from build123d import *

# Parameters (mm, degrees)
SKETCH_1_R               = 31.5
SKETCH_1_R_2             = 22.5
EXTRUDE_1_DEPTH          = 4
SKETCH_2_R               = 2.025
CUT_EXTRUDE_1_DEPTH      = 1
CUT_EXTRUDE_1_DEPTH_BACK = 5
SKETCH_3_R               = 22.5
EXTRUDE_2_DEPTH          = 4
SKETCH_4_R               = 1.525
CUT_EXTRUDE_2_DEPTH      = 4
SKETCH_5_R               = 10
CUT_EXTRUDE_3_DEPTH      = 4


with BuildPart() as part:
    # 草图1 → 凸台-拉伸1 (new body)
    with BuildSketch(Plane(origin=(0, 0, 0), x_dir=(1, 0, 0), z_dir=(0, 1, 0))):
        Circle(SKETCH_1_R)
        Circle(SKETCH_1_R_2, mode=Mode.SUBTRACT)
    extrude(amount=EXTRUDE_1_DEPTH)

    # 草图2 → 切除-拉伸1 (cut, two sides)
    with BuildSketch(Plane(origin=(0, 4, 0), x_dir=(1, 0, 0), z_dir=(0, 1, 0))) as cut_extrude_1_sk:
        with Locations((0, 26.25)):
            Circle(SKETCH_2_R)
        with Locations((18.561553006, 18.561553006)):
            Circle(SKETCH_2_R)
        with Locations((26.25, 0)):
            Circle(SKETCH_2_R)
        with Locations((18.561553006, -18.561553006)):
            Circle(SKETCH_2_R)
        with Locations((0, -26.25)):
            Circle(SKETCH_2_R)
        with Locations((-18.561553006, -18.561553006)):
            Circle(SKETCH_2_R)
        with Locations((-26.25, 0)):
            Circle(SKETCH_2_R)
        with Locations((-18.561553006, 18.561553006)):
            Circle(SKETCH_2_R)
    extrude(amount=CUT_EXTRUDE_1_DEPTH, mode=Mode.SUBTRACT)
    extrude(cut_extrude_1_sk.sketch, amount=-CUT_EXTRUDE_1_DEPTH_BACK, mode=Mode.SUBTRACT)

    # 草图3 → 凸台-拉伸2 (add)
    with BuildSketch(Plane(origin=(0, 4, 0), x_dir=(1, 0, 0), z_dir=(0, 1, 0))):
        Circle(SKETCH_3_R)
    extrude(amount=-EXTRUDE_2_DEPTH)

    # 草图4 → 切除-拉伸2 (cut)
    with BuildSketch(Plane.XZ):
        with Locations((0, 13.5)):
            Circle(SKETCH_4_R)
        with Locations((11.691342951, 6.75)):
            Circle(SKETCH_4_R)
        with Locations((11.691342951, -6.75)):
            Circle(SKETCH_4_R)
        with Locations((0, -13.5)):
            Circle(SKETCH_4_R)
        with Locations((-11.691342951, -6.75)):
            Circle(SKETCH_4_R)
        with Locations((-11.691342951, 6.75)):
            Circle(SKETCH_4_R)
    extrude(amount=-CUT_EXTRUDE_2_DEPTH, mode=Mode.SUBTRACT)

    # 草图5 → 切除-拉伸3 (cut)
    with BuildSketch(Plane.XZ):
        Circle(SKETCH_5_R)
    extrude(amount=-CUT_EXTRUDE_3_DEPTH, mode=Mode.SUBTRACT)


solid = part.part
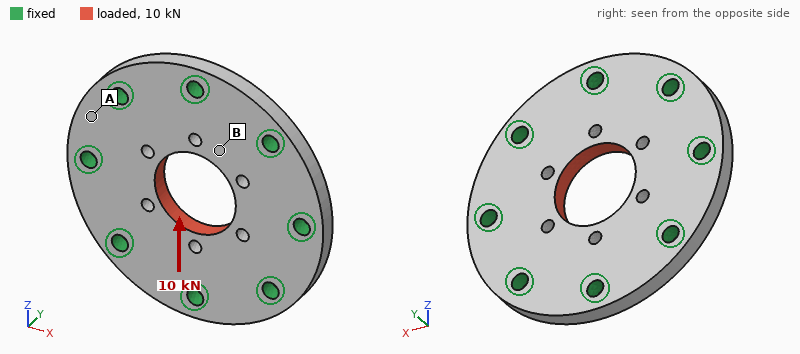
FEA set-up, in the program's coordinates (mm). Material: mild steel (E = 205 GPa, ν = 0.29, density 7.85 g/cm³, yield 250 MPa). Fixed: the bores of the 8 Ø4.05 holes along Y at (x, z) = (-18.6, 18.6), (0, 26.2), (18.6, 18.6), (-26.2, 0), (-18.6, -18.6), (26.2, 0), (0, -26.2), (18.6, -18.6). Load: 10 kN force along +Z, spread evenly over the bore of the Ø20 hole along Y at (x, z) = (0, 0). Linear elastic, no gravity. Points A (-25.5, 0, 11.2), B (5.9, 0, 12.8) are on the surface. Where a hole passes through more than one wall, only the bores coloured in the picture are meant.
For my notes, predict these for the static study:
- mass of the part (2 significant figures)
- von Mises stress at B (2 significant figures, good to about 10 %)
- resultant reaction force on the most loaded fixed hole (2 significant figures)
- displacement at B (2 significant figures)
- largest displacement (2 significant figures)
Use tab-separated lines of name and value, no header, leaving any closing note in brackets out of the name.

mass of the part	83 g
von Mises stress at B	33 MPa
resultant reaction force on the most loaded fixed hole	2.0 kN
displacement at B	2.5 µm
largest displacement	4.2 µm
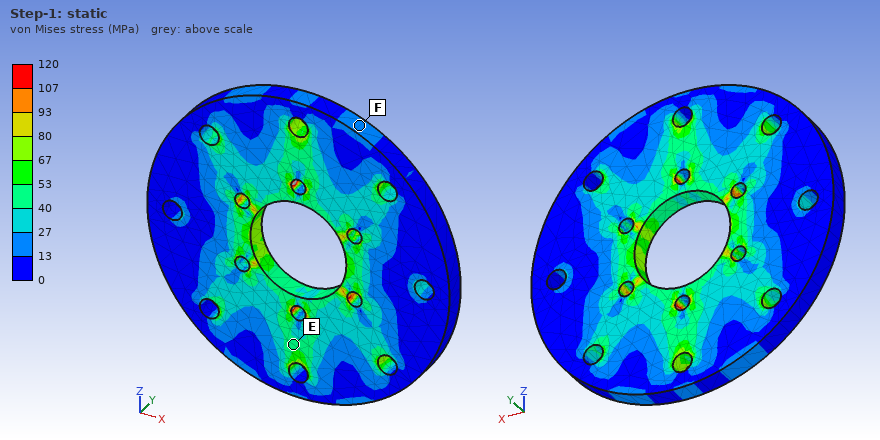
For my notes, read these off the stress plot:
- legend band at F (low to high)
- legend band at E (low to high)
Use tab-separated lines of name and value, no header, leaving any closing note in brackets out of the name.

legend band at F	13 to 27 MPa
legend band at E	40 to 53 MPa
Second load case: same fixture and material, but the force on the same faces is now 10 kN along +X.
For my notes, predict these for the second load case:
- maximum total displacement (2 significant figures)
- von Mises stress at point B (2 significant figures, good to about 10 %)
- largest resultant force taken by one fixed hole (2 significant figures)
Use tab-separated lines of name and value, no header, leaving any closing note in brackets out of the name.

maximum total displacement	4.0 µm
von Mises stress at point B	38 MPa
largest resultant force taken by one fixed hole	2.0 kN
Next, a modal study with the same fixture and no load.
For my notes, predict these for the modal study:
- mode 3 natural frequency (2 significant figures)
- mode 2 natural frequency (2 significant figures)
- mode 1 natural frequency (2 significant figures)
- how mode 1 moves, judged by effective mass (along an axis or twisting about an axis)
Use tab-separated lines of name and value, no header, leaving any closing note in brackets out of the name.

mode 3 natural frequency	23 kHz
mode 2 natural frequency	23 kHz
mode 1 natural frequency	17 kHz
how mode 1 moves, judged by effective mass	along Y
